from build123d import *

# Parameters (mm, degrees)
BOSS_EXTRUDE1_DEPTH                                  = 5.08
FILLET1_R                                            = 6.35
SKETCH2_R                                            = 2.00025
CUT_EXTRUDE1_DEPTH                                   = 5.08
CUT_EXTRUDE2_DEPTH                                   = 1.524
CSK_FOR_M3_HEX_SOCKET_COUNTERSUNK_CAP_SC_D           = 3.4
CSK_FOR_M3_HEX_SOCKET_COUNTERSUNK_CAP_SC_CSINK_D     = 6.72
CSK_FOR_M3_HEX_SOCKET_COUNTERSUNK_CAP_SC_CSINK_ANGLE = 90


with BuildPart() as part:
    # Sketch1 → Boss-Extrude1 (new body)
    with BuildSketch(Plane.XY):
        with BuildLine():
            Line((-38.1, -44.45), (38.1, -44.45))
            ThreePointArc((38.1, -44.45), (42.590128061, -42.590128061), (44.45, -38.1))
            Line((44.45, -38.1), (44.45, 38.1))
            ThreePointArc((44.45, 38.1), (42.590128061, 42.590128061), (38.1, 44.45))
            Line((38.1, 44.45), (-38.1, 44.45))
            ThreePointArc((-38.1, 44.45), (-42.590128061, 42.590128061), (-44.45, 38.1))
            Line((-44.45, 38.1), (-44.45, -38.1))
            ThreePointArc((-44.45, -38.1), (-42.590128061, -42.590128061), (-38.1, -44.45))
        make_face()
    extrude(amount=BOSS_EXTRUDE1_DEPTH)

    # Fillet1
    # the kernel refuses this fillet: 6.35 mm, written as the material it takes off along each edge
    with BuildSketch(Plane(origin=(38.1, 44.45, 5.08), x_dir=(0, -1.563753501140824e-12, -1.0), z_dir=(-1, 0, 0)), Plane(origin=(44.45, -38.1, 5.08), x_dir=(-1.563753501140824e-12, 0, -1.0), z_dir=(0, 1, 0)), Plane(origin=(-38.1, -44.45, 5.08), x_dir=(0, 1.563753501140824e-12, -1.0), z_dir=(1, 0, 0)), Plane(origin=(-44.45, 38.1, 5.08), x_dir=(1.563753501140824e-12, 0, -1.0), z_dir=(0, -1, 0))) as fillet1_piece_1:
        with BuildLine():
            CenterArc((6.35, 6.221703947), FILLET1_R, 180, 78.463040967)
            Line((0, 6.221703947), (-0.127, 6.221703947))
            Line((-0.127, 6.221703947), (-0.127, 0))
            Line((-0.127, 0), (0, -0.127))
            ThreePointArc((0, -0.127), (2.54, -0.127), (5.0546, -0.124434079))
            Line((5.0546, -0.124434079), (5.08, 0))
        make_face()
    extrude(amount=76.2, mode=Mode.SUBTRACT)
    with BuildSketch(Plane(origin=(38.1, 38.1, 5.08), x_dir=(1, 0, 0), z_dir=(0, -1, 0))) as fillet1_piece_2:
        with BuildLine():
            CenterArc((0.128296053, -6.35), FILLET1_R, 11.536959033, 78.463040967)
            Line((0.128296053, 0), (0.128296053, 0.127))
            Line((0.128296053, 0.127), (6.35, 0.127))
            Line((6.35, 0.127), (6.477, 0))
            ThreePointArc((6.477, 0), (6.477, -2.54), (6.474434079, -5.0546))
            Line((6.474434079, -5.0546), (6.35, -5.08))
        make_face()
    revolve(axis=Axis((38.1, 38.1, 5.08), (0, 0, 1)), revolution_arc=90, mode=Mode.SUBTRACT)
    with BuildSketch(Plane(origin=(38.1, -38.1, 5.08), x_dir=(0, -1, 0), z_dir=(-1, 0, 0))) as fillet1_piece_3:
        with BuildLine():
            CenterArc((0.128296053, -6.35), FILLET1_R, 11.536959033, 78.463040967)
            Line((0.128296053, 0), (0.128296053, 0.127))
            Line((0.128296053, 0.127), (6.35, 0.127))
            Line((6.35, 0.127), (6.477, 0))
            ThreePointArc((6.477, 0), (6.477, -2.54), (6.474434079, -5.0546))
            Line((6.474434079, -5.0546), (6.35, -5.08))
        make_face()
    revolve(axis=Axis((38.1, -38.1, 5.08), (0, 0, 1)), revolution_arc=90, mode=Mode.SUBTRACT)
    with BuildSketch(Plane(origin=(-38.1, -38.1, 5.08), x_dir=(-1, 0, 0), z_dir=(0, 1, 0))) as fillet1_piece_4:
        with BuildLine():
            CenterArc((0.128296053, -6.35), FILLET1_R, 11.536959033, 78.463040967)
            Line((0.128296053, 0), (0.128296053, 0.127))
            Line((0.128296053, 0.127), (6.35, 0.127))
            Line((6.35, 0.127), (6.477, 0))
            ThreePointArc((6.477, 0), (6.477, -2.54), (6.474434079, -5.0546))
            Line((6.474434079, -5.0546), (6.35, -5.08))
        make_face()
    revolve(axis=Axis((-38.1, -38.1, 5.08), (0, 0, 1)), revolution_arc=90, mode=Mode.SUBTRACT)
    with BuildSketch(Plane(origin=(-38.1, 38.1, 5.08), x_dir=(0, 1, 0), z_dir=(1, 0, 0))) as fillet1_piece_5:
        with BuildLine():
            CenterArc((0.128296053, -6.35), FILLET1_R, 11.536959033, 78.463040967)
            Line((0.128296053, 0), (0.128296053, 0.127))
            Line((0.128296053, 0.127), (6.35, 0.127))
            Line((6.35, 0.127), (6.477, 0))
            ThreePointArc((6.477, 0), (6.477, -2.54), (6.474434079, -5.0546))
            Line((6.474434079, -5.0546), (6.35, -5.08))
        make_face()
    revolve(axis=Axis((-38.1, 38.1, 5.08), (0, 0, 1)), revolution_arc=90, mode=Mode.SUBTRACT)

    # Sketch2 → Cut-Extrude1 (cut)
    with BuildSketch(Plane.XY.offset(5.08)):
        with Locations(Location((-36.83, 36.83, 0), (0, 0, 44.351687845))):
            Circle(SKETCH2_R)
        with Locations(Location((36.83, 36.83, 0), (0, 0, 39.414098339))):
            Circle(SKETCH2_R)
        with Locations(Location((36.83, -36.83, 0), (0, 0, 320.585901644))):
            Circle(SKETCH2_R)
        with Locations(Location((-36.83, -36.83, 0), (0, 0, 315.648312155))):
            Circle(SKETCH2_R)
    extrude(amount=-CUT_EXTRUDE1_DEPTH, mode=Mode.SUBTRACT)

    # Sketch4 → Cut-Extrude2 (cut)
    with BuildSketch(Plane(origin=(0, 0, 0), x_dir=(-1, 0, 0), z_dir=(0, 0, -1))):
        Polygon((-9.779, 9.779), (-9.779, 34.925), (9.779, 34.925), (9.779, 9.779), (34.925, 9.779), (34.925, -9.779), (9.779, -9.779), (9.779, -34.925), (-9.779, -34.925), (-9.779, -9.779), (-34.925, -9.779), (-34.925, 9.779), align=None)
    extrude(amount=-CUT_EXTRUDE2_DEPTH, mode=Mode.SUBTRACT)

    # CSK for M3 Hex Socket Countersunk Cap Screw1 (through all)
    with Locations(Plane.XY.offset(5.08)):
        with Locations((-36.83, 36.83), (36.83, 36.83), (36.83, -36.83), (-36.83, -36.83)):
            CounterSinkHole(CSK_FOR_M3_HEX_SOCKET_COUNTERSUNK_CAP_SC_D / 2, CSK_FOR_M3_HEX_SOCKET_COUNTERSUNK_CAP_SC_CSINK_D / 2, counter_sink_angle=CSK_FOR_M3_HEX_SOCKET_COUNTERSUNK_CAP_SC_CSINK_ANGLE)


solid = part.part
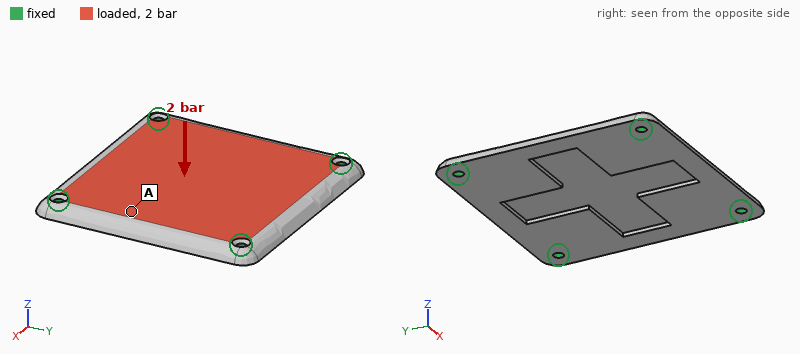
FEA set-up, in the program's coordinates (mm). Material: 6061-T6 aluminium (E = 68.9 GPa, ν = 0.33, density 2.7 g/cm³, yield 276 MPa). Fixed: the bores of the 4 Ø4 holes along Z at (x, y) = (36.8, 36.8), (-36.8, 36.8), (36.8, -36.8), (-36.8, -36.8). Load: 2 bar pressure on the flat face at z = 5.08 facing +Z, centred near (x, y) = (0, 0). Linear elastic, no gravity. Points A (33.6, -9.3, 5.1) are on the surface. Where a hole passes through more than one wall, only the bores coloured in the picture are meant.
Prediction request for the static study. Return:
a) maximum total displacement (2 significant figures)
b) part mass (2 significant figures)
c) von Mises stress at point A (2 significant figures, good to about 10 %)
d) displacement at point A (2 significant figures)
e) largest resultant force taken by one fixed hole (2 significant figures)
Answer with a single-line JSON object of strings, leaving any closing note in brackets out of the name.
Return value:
{"maximum total displacement": "92 µm", "part mass": "90 g", "von Mises stress at point A": "15 MPa", "displacement at point A": "42 µm", "largest resultant force taken by one fixed hole": "490 N"}
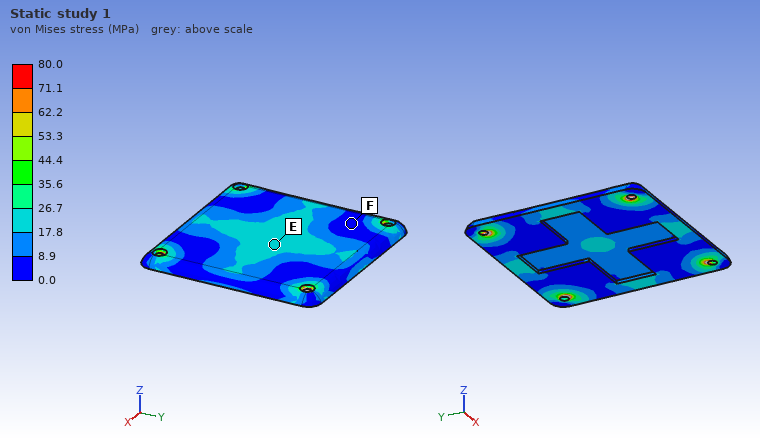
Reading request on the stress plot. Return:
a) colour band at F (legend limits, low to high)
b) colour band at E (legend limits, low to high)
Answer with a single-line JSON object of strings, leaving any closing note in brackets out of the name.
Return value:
{"colour band at F": "0.0 to 8.9 MPa", "colour band at E": "17.8 to 26.7 MPa"}
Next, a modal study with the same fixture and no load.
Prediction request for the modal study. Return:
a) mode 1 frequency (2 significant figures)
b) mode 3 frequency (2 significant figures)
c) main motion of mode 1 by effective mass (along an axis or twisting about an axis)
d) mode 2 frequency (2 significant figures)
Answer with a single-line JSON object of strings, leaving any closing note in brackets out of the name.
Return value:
{"mode 1 frequency": "2700 Hz", "mode 3 frequency": "4600 Hz", "main motion of mode 1 by effective mass": "along Z", "mode 2 frequency": "4600 Hz"}
